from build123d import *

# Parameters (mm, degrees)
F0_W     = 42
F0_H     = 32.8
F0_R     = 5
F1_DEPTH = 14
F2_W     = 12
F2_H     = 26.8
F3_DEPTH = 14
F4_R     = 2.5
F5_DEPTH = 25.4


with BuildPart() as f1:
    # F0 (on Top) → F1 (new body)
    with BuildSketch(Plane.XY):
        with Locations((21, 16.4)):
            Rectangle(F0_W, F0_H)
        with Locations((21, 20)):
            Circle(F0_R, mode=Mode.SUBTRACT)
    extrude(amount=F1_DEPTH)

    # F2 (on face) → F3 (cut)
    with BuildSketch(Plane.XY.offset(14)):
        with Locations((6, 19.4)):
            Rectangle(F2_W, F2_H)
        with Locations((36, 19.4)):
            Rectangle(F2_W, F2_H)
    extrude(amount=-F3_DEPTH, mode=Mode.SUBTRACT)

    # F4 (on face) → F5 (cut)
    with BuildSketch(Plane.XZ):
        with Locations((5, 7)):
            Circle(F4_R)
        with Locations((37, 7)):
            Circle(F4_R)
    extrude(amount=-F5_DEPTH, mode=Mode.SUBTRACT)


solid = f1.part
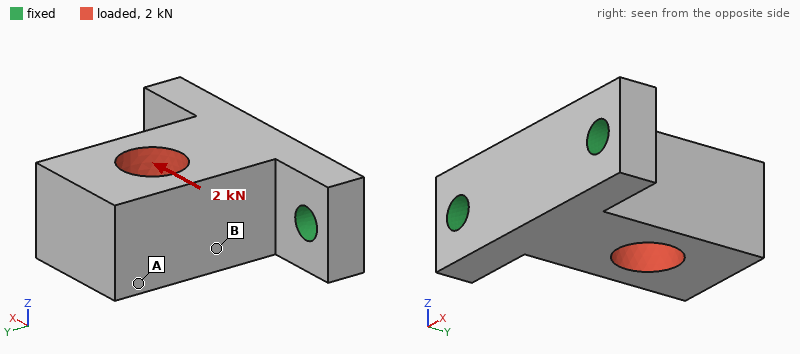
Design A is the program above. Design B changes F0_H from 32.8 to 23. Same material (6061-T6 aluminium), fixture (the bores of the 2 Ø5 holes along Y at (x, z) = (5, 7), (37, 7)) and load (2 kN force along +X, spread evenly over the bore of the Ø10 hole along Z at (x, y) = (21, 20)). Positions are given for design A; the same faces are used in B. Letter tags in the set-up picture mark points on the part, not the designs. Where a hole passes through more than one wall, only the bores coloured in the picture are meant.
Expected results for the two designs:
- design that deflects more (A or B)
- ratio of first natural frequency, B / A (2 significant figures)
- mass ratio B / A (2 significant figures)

B
0.25
0.56
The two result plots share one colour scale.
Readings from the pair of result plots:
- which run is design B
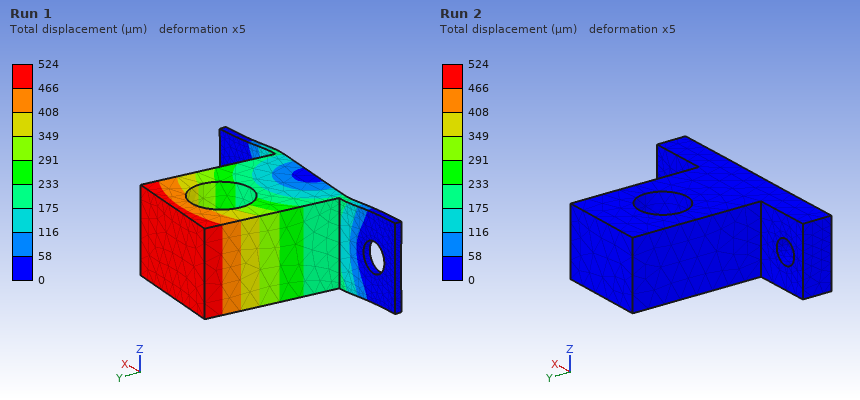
Run 1
